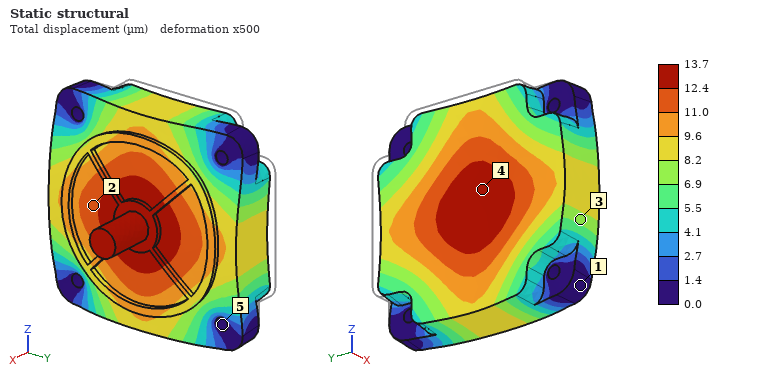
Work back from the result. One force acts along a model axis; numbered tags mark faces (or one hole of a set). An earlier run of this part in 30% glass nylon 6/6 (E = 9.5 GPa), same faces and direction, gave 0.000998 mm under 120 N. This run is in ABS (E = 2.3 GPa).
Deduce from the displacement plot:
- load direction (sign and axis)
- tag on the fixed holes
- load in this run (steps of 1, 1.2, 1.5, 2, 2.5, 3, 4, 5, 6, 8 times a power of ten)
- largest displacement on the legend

+X
5
400 N
13.7 µm
